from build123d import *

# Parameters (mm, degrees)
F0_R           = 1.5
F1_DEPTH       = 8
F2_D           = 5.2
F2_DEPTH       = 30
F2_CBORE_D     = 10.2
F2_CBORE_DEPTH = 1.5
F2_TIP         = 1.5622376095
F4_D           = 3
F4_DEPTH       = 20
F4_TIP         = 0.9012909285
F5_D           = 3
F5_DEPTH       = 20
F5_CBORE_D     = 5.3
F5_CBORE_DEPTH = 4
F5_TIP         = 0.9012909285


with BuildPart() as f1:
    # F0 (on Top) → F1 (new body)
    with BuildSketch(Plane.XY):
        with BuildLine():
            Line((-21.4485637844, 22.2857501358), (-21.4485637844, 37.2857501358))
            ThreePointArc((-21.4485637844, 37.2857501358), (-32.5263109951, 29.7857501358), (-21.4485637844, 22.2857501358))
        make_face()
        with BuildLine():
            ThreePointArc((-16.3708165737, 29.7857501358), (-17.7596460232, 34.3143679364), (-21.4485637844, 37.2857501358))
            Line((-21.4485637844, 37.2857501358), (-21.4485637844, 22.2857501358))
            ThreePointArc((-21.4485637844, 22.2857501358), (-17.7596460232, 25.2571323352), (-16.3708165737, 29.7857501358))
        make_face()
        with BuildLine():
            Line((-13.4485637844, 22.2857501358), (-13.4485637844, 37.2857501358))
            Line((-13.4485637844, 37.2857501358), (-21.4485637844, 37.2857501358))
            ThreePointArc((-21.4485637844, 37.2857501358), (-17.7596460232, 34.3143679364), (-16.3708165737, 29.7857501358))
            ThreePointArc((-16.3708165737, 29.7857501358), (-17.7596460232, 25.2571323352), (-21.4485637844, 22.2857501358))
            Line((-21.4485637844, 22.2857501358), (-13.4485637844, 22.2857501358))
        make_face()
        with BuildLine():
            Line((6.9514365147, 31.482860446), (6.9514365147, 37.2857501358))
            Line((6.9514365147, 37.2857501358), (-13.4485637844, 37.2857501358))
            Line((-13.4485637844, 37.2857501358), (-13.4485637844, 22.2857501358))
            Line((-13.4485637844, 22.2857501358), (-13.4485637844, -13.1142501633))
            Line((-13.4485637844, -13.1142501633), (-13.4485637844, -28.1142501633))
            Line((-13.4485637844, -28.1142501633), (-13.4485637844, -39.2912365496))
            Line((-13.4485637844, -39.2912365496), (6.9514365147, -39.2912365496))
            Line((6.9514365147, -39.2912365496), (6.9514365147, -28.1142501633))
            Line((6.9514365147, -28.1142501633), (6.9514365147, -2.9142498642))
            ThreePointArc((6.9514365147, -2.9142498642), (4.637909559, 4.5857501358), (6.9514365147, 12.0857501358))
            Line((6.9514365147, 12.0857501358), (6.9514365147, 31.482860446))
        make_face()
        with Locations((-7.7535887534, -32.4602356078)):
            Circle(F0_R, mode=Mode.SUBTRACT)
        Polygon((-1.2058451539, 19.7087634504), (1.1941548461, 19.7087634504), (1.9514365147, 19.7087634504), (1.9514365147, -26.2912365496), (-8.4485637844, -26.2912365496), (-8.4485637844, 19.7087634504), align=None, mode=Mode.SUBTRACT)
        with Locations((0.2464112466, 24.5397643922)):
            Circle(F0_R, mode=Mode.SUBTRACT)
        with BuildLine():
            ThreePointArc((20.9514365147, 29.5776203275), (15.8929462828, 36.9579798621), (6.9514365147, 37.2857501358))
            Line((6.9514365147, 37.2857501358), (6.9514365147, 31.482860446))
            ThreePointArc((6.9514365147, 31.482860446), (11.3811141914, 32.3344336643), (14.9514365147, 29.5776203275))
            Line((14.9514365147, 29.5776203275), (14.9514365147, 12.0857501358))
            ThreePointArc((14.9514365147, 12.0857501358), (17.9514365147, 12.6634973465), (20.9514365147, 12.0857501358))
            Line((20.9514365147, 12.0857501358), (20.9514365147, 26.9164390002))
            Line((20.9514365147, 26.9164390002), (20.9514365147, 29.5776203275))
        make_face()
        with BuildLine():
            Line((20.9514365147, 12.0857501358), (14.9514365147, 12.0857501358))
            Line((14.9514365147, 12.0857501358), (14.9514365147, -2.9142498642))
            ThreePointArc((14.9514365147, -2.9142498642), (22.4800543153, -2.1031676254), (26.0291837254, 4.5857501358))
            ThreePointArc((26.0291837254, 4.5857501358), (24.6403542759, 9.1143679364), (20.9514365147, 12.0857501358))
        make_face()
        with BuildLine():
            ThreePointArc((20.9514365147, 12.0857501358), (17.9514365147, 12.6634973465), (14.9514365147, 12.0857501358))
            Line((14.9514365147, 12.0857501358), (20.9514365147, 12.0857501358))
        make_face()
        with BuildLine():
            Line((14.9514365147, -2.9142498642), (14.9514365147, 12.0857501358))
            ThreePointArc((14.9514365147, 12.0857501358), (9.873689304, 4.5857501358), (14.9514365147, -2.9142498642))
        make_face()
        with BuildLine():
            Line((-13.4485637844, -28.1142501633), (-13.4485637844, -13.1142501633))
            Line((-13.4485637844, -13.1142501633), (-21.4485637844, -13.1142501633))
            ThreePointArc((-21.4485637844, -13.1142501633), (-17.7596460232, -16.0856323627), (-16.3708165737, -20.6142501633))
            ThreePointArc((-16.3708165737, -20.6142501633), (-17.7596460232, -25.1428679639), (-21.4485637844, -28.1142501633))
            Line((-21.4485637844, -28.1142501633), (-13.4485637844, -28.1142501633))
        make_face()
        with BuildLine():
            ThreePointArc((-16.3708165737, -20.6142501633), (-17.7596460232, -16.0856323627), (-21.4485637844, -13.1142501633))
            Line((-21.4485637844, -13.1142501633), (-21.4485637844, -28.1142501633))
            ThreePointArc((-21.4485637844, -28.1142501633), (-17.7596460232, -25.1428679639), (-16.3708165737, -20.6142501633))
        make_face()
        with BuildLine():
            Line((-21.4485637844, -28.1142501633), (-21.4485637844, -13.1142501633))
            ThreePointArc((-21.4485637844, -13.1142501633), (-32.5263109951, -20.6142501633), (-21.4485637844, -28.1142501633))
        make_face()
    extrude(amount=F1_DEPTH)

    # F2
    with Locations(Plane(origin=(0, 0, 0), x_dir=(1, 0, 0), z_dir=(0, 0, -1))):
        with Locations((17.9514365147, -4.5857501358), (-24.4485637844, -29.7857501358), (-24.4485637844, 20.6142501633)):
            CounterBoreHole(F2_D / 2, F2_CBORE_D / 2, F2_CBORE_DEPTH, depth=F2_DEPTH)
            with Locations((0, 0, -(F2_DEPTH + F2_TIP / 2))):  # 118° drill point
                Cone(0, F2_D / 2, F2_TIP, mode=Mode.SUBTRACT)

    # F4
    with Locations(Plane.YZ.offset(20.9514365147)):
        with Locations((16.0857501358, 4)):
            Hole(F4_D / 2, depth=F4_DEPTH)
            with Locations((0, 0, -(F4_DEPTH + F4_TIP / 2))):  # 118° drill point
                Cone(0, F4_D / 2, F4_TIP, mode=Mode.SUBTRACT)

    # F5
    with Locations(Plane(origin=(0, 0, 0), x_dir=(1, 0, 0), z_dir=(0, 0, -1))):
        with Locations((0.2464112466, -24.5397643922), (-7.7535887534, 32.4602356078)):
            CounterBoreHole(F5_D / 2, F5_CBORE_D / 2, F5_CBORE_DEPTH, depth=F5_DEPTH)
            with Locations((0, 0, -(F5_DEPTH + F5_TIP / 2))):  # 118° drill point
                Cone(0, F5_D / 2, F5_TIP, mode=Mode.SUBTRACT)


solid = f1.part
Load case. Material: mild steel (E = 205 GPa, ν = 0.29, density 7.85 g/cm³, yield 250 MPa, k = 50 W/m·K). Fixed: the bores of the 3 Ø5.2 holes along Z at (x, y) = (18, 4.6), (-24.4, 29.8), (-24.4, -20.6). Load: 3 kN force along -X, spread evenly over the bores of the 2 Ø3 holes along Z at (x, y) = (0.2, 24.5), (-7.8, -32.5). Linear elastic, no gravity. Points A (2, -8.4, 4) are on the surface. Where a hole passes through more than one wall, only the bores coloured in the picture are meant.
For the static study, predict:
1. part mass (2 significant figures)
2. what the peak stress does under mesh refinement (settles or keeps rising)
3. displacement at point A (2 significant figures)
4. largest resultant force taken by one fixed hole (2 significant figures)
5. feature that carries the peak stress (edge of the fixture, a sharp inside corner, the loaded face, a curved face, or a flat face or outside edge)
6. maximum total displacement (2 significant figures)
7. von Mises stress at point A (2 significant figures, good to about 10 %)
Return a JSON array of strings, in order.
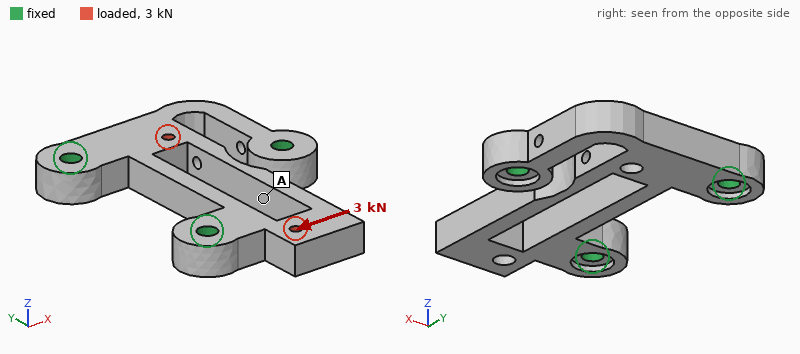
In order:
["120 g", "keeps rising", "11 µm", "1.6 kN", "a sharp inside corner", "22 µm", "10 MPa"]
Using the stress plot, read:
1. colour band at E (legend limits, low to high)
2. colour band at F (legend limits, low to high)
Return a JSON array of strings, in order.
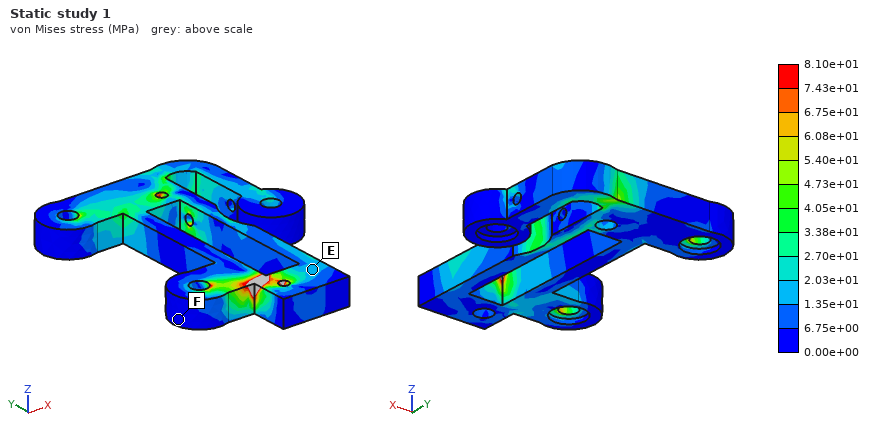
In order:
["1.35e+01 to 2.03e+01 MPa", "0.00e+00 to 6.75e+00 MPa"]
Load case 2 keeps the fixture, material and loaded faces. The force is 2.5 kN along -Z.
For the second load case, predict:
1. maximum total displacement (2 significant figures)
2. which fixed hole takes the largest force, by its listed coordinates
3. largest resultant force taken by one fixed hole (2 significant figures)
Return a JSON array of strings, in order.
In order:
["88 µm", "(-24.4, -20.6)", "1.4 kN"]
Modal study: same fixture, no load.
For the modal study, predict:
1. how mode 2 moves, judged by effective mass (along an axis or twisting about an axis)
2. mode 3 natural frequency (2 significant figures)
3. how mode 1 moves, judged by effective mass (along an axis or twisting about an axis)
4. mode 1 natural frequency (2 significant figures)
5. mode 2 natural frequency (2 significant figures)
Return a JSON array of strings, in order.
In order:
["along Z", "8000 Hz", "along Z", "4100 Hz", "5900 Hz"]
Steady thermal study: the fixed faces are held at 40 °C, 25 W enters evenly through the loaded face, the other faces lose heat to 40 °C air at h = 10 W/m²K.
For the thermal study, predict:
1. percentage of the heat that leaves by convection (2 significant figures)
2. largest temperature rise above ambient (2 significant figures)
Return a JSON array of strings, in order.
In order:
["8.1 %", "71 K"]
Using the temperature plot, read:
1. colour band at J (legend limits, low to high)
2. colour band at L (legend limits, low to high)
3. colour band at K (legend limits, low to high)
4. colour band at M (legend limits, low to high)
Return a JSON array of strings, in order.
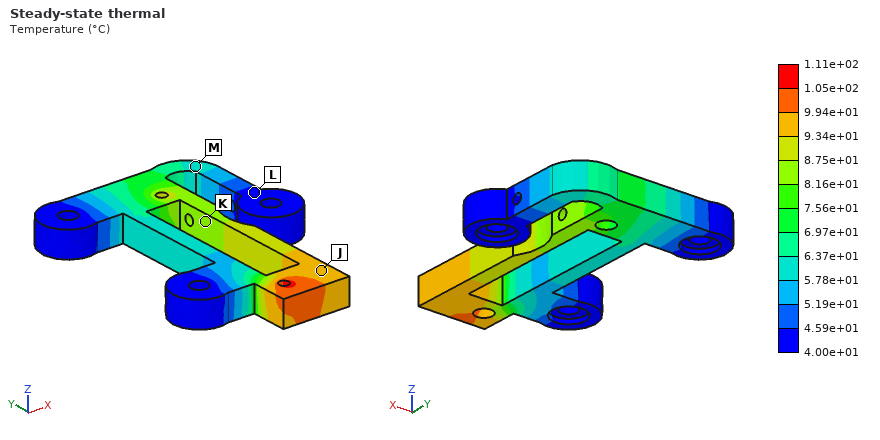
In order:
["9.34e+01 to 9.94e+01 °C", "4.00e+01 to 4.59e+01 °C", "8.16e+01 to 8.75e+01 °C", "5.78e+01 to 6.37e+01 °C"]
